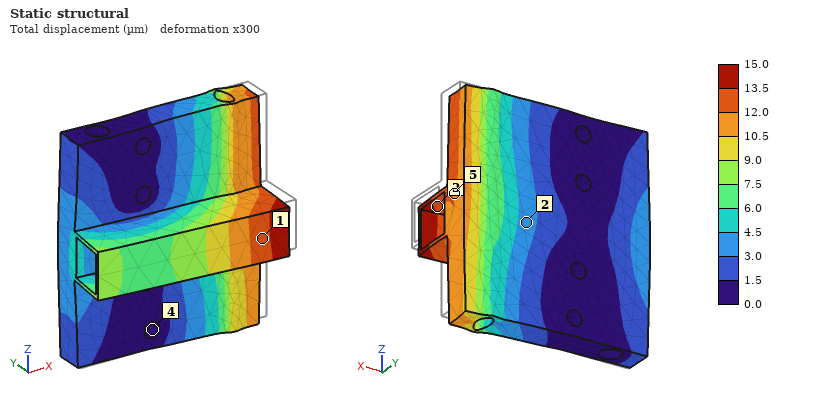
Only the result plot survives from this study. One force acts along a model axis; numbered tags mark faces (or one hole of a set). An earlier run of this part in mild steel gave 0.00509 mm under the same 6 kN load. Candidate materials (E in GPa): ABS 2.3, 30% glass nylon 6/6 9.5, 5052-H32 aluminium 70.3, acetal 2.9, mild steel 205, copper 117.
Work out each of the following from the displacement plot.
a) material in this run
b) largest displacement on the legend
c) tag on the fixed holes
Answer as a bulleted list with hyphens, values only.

- 5052-H32 aluminium
- 15.0 µm
- 4
